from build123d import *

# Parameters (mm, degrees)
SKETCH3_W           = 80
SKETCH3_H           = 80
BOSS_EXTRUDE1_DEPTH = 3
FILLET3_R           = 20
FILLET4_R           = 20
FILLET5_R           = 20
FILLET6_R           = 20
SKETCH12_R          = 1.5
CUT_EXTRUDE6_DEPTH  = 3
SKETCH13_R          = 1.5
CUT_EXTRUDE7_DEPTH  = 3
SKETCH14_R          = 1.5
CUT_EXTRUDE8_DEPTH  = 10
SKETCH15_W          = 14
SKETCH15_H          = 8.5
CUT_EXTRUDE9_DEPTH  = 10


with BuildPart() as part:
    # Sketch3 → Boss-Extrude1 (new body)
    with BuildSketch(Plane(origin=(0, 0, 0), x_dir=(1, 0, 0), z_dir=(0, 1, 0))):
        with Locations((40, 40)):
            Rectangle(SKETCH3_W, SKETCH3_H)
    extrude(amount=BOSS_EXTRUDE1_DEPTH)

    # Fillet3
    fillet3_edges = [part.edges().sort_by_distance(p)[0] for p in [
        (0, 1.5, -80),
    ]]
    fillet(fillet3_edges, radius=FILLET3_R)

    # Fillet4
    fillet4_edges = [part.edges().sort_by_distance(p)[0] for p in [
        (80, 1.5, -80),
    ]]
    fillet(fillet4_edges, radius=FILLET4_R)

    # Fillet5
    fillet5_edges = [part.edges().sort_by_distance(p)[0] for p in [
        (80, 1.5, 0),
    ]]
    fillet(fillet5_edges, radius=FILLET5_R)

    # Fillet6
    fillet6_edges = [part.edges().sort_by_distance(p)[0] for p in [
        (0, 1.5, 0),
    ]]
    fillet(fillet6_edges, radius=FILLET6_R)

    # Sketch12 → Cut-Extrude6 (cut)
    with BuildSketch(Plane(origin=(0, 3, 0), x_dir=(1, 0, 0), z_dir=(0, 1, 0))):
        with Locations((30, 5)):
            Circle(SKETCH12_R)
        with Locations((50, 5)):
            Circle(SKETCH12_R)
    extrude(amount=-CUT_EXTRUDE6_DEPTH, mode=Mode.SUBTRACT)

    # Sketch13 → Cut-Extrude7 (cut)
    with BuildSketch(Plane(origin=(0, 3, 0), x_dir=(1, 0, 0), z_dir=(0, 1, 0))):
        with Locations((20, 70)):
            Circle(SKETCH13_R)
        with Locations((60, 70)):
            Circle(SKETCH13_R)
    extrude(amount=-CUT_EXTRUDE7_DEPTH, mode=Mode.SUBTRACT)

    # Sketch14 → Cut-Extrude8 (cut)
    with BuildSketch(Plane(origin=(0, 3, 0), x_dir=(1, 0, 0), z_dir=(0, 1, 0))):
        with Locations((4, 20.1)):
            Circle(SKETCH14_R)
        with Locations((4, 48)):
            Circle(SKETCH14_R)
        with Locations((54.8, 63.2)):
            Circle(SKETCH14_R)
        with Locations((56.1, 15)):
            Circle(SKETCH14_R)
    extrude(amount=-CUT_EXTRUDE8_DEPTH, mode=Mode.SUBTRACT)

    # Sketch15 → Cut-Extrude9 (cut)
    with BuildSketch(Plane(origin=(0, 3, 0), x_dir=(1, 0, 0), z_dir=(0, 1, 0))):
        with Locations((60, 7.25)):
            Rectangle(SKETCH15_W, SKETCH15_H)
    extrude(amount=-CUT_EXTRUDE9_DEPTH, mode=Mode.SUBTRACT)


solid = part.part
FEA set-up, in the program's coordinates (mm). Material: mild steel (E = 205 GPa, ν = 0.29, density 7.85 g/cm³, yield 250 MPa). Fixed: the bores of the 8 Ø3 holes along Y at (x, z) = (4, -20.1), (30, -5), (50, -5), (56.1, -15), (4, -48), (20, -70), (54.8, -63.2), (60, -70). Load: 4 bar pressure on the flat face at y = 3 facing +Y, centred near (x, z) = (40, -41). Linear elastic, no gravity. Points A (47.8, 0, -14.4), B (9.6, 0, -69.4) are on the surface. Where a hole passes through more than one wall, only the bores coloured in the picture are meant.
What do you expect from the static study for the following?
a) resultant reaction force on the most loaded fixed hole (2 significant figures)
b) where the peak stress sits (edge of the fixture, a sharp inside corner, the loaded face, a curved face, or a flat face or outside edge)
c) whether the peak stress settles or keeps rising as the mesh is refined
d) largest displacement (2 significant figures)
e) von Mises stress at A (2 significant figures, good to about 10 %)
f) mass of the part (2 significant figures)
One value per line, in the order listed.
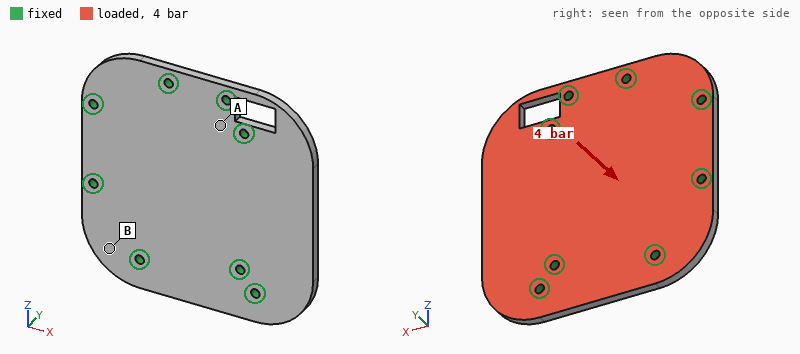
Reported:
570 N
edge of the fixture
keeps rising
59 µm
23 MPa
140 g
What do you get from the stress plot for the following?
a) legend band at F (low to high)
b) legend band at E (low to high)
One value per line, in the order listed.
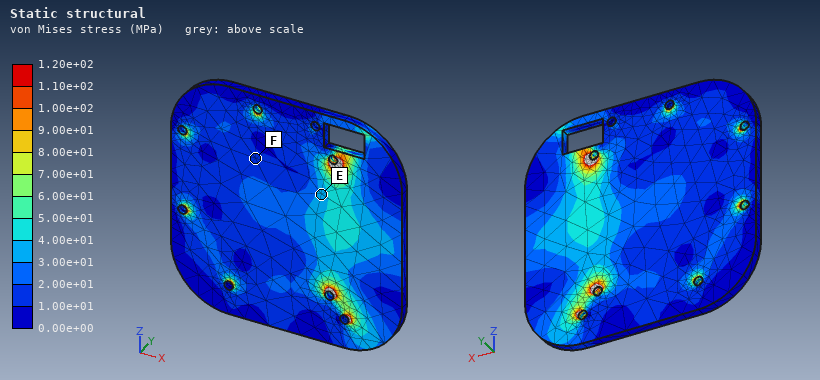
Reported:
1.00e+01 to 2.00e+01 MPa
3.00e+01 to 4.00e+01 MPa
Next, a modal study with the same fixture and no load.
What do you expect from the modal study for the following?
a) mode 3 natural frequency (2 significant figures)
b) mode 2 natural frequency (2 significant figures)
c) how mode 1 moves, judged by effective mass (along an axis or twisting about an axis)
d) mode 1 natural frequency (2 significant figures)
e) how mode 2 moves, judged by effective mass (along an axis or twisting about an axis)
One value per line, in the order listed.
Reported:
6200 Hz
5400 Hz
along Y
3500 Hz
along Y
